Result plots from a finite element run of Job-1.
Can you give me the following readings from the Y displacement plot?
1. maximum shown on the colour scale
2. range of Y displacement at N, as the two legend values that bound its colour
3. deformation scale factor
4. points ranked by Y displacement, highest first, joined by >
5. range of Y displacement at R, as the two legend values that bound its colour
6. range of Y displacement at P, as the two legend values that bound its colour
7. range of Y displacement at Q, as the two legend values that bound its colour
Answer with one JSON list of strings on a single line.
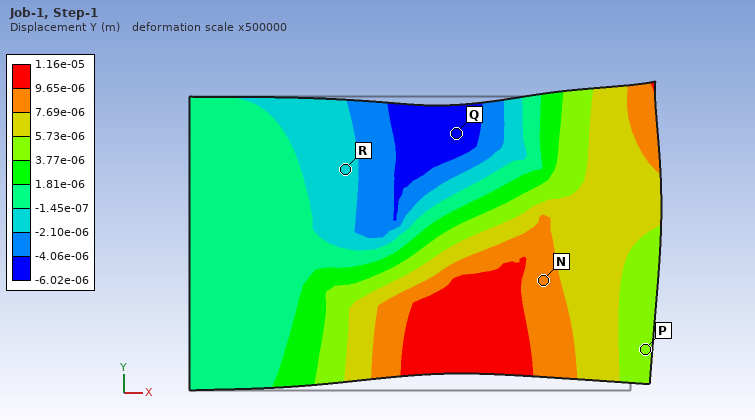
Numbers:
["1.16e-05 m", "7.69e-06 to 9.65e-06 m", "500000", "N > P > R > Q", "-2.10e-06 to -1.45e-07 m", "3.77e-06 to 5.73e-06 m", "-6.02e-06 to -4.06e-06 m"]
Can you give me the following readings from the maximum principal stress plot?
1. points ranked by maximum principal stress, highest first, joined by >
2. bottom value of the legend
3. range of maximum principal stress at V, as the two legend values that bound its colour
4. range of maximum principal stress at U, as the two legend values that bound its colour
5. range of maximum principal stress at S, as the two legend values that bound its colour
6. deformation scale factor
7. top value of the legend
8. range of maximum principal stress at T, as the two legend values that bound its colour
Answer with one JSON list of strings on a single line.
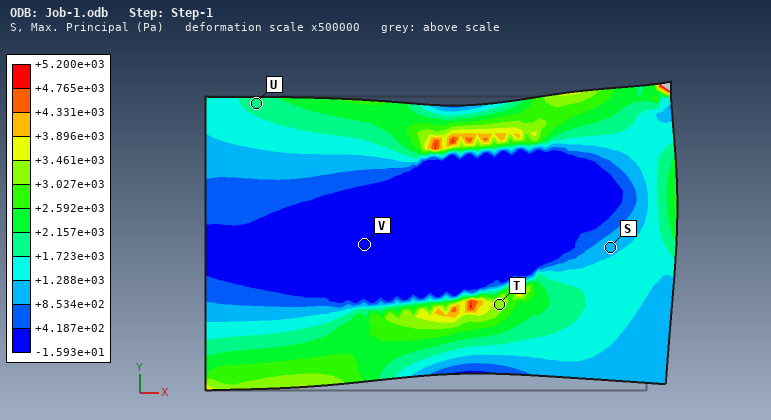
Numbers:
["T > U > S > V", "-1.593e+01 Pa", "-1.593e+01 to +4.187e+02 Pa", "+1.723e+03 to +2.157e+03 Pa", "+8.534e+02 to +1.288e+03 Pa", "500000", "+5.200e+03 Pa", "+3.027e+03 to +3.461e+03 Pa"]
